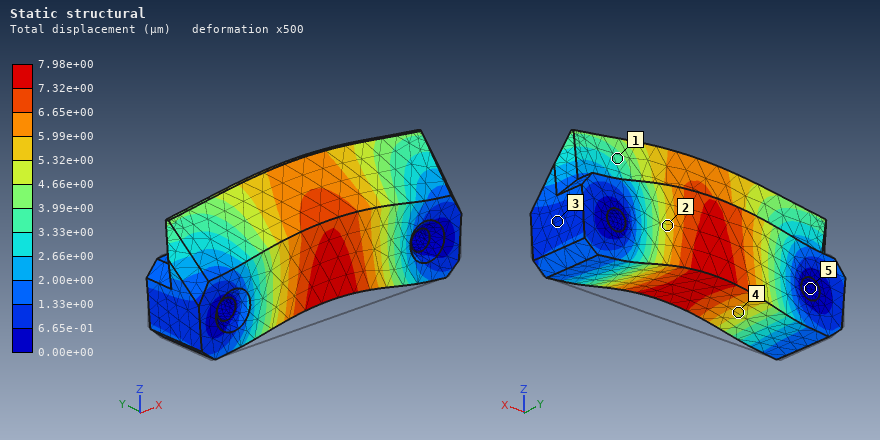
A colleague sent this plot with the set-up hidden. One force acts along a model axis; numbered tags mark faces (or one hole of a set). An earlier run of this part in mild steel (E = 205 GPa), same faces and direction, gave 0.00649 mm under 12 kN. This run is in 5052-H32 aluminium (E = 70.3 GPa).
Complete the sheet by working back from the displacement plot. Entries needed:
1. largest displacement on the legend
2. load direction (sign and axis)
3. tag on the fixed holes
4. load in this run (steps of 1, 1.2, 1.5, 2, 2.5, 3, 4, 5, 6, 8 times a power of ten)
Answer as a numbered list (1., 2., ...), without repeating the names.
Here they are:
1. 7.98e+00 µm
2. +Z
3. 5
4. 5 kN
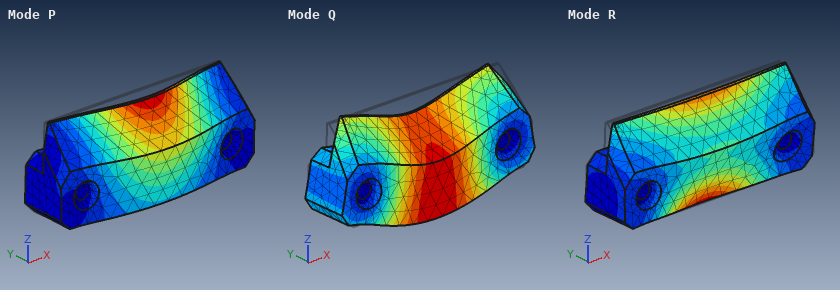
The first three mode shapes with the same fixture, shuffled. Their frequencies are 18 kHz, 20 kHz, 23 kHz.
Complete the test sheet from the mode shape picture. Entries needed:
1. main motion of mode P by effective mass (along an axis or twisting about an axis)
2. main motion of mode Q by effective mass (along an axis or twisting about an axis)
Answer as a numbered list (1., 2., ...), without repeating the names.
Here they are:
1. along Y
2. along Z
